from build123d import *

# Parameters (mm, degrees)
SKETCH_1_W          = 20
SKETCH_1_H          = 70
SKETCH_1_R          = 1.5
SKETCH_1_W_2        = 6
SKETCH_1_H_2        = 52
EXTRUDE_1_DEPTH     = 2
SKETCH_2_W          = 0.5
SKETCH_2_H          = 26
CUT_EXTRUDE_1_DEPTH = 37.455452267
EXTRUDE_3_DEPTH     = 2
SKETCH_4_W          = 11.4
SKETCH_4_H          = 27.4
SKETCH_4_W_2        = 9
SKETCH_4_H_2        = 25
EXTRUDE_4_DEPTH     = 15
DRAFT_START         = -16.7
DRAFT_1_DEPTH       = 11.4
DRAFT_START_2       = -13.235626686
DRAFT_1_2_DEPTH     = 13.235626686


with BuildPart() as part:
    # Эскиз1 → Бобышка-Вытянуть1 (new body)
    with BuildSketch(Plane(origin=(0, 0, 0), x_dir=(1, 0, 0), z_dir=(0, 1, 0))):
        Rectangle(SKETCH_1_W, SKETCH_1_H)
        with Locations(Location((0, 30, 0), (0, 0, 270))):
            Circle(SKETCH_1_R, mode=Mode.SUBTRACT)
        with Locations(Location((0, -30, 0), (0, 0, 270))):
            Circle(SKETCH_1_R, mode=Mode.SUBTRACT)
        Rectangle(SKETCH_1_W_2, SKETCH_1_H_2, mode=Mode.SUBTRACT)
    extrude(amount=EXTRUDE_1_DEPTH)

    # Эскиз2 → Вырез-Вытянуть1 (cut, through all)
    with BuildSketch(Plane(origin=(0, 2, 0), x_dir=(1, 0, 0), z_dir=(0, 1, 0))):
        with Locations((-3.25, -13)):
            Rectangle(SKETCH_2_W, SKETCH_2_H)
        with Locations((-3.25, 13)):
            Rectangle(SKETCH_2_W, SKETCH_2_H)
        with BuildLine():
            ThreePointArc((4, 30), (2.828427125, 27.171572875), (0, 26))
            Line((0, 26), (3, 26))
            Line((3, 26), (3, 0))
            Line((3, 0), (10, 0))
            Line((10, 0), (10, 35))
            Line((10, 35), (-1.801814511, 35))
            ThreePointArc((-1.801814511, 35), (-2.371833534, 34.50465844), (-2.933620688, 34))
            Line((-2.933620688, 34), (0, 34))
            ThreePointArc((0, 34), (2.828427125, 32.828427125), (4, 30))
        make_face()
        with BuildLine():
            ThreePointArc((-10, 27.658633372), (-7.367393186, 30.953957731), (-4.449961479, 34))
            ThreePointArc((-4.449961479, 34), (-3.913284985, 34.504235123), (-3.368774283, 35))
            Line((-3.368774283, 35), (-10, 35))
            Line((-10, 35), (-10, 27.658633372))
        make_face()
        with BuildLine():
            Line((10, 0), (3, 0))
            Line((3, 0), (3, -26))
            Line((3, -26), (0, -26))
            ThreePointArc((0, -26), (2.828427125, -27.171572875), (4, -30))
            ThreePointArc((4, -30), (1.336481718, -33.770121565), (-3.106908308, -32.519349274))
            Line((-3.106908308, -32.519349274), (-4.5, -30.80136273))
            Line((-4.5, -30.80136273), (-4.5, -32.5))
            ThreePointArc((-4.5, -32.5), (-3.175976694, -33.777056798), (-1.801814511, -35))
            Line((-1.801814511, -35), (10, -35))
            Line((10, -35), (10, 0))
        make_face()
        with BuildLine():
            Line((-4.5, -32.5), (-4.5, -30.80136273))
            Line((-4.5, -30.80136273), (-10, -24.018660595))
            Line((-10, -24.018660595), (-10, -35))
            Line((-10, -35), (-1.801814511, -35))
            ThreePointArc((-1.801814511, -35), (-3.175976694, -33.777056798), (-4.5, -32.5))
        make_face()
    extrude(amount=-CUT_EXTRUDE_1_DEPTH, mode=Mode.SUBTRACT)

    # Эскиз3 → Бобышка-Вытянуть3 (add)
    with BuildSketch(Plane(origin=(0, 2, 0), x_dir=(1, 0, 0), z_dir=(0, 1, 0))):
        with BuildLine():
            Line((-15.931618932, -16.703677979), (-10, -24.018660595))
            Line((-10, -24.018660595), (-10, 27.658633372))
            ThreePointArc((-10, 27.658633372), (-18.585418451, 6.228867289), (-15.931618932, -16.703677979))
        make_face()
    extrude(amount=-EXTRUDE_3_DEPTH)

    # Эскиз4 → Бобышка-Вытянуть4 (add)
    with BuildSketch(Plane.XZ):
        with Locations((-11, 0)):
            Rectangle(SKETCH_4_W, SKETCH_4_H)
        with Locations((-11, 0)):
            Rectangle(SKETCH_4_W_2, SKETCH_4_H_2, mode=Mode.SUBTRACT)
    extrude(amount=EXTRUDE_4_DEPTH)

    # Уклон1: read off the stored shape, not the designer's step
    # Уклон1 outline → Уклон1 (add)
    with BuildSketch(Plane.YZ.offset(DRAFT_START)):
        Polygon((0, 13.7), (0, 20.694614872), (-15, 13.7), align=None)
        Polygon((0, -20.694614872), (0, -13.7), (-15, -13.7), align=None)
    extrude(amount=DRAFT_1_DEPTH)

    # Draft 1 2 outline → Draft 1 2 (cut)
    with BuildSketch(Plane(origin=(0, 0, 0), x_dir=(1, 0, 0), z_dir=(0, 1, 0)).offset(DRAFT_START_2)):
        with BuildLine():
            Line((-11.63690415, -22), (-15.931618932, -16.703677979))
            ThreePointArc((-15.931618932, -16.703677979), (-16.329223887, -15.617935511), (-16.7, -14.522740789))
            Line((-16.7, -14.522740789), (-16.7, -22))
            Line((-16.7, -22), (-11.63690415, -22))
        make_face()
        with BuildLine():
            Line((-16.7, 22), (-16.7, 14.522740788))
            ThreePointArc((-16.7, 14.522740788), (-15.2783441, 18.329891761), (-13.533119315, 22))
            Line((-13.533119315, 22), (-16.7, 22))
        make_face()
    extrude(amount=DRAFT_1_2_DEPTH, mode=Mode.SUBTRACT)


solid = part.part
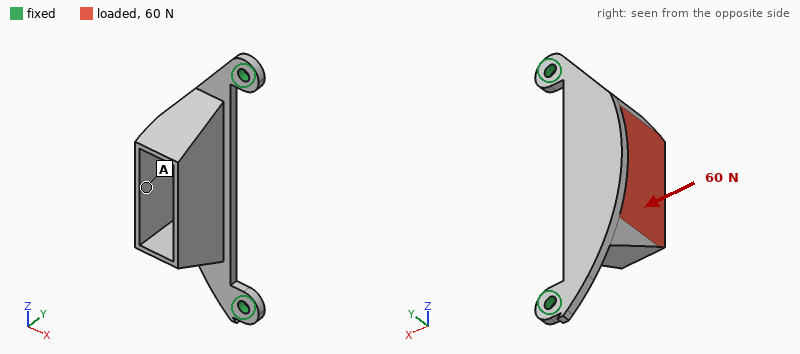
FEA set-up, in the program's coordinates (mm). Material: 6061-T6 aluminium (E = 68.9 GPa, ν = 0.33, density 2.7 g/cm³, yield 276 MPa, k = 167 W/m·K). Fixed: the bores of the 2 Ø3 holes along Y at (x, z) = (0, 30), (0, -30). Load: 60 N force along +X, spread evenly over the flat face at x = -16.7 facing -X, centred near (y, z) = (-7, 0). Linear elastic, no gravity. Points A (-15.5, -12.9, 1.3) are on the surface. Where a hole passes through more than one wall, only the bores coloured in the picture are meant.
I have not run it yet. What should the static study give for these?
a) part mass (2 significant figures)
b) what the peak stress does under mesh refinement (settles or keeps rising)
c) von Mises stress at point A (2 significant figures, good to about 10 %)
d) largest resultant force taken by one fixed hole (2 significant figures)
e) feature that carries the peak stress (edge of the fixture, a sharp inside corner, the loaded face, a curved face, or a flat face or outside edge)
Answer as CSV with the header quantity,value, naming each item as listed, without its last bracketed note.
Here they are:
quantity,value
part mass,11 g
what the peak stress does under mesh refinement,keeps rising
von Mises stress at point A,11 MPa
largest resultant force taken by one fixed hole,42 N
feature that carries the peak stress,a sharp inside corner
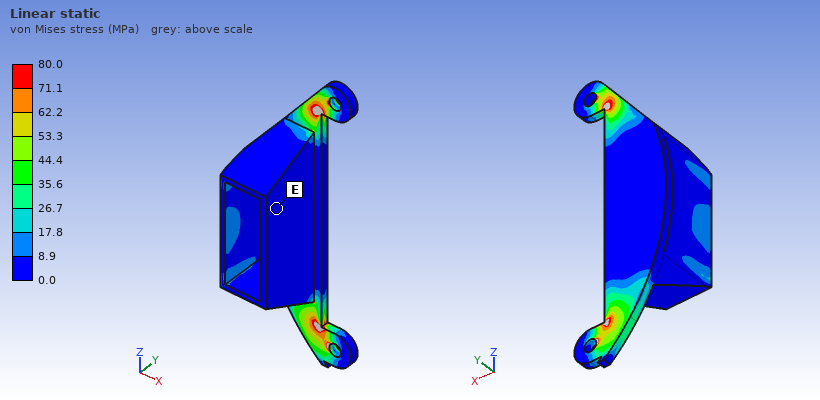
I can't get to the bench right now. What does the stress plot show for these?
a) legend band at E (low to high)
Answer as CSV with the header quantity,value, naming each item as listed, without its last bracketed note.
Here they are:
quantity,value
legend band at E,0.0 to 8.9 MPa
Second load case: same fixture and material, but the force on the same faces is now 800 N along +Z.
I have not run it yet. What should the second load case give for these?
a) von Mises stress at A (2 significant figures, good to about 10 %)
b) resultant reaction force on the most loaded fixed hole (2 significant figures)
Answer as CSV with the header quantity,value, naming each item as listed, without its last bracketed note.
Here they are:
quantity,value
von Mises stress at A,19 MPa
resultant reaction force on the most loaded fixed hole,460 N
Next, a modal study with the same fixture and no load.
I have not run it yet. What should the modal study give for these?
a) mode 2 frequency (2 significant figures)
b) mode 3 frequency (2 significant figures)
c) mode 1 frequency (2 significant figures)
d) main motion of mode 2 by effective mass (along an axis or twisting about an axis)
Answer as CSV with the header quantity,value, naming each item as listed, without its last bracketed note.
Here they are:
quantity,value
mode 2 frequency,3800 Hz
mode 3 frequency,4900 Hz
mode 1 frequency,1200 Hz
main motion of mode 2 by effective mass,along Y
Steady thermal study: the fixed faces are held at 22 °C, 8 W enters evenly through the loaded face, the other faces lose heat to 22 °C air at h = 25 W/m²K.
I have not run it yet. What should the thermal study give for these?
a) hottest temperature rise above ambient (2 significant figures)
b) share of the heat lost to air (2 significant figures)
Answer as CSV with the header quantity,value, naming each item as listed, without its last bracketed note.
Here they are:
quantity,value
hottest temperature rise above ambient,28 K
share of the heat lost to air,23 %
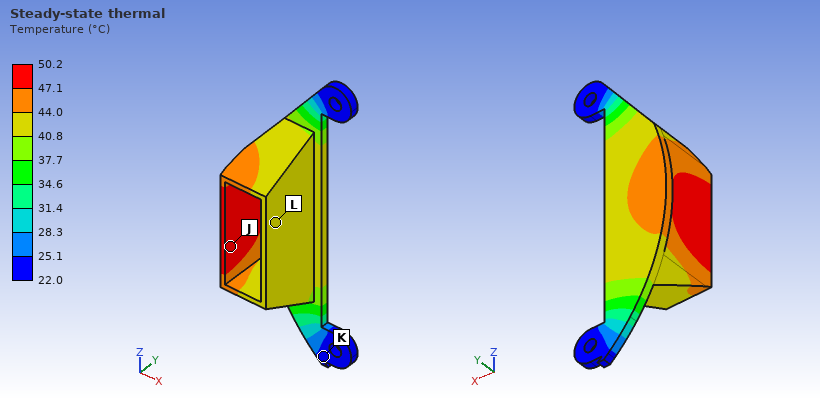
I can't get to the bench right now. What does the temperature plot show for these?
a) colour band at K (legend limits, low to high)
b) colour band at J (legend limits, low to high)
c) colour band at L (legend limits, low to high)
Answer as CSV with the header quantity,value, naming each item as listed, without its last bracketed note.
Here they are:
quantity,value
colour band at K,22.0 to 25.1 °C
colour band at J,47.1 to 50.2 °C
colour band at L,40.8 to 44.0 °C
